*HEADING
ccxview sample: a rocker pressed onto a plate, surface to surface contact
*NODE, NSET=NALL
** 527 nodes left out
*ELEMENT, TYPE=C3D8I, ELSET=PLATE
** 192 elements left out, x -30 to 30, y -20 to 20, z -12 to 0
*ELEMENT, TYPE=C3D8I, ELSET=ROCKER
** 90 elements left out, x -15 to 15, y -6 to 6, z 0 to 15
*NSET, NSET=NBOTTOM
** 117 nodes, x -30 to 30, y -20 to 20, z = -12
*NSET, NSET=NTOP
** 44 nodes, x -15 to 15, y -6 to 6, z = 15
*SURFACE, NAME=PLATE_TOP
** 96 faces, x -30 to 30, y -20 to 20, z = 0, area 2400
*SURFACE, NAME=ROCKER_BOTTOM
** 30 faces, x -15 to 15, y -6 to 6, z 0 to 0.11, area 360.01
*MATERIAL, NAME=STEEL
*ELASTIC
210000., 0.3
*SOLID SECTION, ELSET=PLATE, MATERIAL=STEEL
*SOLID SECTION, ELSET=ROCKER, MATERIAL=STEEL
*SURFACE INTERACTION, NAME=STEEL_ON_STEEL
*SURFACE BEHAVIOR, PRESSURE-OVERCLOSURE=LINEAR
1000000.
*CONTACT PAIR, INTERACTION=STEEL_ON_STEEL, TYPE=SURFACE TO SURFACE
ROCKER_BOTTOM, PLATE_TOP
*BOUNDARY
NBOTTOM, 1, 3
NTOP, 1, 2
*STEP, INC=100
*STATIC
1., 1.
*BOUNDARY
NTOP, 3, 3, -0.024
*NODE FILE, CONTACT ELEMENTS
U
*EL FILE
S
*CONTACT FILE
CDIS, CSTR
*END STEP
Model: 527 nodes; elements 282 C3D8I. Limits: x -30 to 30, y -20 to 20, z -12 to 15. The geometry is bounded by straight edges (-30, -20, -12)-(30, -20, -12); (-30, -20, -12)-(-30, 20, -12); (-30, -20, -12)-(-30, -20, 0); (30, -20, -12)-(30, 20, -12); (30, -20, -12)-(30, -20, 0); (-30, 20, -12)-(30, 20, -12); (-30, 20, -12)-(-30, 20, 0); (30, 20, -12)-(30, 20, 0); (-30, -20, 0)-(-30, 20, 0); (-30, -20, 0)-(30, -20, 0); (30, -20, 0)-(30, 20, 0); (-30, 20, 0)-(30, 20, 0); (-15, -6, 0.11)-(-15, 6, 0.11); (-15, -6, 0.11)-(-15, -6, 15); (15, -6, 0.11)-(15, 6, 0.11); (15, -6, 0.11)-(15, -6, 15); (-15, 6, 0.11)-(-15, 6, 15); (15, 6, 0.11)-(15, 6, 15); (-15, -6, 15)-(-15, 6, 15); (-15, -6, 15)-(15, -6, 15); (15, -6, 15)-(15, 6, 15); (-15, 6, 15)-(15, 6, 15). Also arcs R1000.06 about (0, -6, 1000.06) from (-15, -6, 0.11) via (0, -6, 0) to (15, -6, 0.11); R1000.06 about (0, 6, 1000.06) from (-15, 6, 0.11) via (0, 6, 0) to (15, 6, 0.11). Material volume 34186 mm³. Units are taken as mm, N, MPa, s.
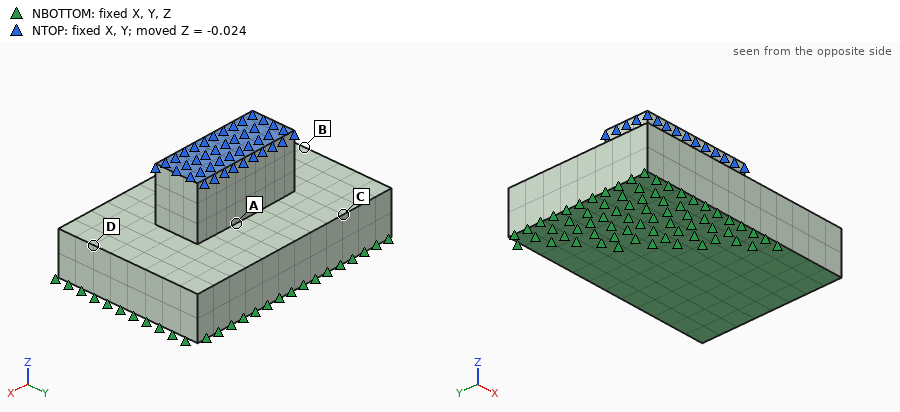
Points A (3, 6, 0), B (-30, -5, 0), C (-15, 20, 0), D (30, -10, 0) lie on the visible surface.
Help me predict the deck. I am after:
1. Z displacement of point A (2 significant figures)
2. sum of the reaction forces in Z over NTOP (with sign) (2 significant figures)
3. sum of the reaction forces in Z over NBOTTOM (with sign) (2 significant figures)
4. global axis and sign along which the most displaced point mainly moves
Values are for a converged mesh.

-0.0099 mm
-30000 N
30000 N
-Z
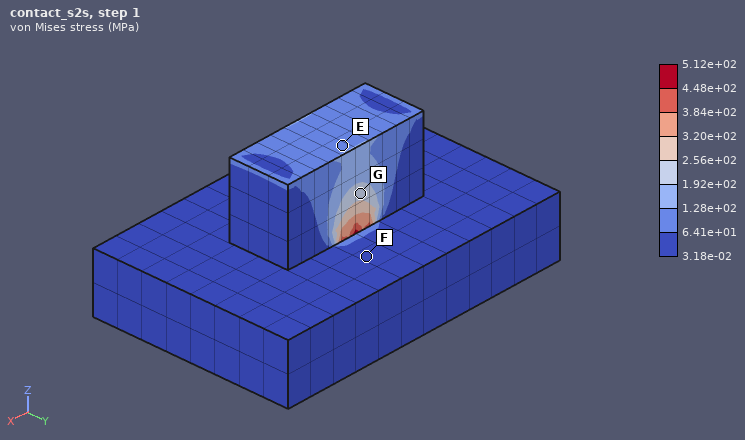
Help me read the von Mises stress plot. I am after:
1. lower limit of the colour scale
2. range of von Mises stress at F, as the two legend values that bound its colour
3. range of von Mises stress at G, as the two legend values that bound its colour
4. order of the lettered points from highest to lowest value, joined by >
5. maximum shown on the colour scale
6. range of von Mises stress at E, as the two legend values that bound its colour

3.18e-02 MPa
3.18e-02 to 6.41e+01 MPa
1.92e+02 to 2.56e+02 MPa
G > E > F
5.12e+02 MPa
6.41e+01 to 1.28e+02 MPa
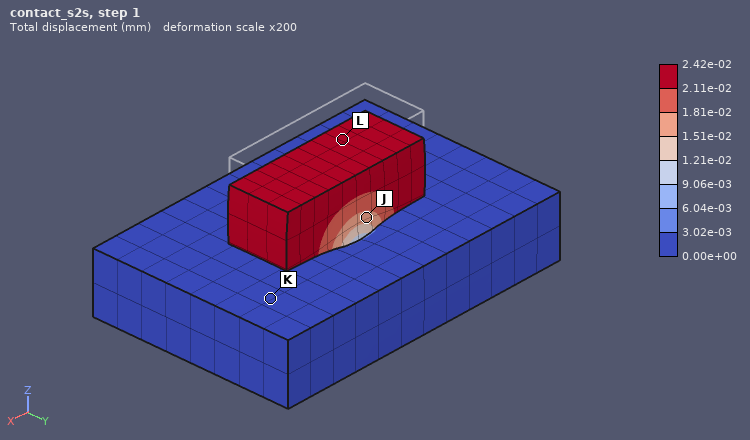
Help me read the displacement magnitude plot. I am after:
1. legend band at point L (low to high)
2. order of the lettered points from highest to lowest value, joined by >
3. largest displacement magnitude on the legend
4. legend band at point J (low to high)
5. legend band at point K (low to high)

2.11e-02 to 2.42e-02 mm
L > J > K
2.42e-02 mm
1.51e-02 to 1.81e-02 mm
0.00e+00 to 3.02e-03 mm
